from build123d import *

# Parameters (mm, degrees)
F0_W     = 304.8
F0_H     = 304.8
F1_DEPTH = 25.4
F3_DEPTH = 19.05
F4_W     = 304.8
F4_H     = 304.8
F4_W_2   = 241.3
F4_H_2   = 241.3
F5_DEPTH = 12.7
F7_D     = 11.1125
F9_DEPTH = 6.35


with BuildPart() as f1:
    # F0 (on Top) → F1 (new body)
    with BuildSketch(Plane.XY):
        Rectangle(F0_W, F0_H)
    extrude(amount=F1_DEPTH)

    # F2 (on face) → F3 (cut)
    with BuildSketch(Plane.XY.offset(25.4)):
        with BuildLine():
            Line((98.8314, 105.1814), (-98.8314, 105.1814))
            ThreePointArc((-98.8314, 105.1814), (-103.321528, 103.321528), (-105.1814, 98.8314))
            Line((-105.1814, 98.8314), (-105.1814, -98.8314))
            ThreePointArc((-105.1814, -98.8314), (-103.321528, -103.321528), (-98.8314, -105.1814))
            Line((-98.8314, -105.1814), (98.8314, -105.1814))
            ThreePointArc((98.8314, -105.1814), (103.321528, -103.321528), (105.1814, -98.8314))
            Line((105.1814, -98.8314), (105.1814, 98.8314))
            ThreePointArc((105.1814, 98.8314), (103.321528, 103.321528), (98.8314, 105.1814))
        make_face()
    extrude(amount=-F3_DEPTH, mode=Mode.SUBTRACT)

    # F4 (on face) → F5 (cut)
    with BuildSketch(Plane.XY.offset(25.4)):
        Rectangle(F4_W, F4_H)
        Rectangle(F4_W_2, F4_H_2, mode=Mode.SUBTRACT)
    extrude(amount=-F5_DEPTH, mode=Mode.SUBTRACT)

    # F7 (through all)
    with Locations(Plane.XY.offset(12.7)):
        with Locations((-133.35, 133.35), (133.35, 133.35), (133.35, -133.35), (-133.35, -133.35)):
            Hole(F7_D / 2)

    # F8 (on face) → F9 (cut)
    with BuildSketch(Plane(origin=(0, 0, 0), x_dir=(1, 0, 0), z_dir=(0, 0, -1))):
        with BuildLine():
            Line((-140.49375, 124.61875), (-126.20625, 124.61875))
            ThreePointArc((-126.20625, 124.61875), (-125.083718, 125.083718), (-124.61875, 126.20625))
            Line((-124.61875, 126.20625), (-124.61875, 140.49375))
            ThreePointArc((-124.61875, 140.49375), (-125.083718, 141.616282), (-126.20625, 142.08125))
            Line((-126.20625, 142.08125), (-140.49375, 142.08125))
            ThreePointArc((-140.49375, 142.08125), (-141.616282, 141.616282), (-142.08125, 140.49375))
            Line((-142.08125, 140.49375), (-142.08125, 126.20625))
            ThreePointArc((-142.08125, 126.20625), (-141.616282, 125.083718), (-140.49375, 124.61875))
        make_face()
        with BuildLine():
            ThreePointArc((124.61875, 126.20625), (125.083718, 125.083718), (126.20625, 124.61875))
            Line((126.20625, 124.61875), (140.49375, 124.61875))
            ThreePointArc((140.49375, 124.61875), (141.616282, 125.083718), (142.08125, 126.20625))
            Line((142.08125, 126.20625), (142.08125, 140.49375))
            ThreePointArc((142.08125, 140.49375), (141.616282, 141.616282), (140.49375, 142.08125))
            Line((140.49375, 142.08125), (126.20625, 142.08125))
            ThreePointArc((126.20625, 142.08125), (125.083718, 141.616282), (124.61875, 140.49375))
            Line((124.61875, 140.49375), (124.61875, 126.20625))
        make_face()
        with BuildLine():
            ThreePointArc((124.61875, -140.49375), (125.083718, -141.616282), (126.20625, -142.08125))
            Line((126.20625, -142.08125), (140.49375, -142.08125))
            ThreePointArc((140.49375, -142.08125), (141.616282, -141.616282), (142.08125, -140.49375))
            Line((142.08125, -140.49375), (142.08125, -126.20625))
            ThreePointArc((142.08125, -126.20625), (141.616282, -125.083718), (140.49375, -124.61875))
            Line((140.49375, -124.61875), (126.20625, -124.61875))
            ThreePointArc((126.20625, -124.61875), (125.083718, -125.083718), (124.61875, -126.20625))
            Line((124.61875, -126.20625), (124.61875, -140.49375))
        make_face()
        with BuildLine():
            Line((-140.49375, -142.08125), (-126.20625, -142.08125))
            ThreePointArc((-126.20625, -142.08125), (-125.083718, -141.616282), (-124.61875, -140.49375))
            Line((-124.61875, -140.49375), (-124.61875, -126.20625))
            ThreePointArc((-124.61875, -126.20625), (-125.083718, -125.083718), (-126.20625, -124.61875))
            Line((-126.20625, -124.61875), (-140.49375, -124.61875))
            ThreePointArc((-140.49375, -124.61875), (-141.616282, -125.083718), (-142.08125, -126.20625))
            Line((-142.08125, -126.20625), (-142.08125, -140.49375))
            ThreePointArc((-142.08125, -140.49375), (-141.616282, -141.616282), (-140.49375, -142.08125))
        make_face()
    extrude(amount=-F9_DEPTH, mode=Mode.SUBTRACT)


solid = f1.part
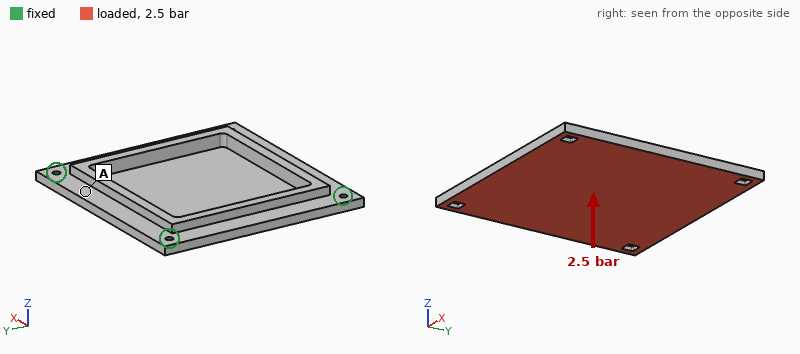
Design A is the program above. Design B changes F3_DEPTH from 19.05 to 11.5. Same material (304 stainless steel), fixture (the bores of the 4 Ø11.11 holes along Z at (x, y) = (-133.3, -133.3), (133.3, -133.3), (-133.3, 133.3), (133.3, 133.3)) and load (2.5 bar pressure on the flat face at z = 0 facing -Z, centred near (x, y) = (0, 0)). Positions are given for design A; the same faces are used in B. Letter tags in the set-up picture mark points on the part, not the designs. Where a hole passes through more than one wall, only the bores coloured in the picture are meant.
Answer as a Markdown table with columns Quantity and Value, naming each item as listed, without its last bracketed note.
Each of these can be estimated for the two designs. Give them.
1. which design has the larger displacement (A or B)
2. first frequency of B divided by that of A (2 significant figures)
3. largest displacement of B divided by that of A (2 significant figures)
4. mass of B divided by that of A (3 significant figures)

| Quantity | Value |
|---|---|
| which design has the larger displacement | A |
| first frequency of B divided by that of A | 0.92 |
| largest displacement of B divided by that of A | 0.53 |
| mass of B divided by that of A | 1.31 |
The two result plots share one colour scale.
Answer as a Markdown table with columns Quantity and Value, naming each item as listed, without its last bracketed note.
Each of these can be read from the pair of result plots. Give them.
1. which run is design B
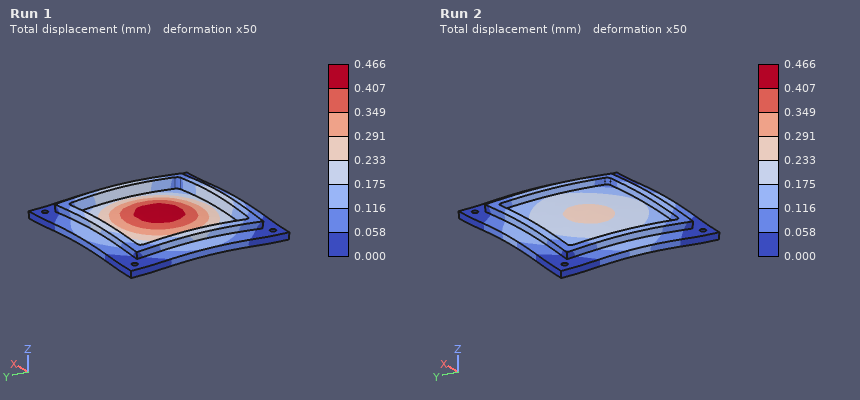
| Quantity | Value |
|---|---|
| which run is design B | Run 2 |
